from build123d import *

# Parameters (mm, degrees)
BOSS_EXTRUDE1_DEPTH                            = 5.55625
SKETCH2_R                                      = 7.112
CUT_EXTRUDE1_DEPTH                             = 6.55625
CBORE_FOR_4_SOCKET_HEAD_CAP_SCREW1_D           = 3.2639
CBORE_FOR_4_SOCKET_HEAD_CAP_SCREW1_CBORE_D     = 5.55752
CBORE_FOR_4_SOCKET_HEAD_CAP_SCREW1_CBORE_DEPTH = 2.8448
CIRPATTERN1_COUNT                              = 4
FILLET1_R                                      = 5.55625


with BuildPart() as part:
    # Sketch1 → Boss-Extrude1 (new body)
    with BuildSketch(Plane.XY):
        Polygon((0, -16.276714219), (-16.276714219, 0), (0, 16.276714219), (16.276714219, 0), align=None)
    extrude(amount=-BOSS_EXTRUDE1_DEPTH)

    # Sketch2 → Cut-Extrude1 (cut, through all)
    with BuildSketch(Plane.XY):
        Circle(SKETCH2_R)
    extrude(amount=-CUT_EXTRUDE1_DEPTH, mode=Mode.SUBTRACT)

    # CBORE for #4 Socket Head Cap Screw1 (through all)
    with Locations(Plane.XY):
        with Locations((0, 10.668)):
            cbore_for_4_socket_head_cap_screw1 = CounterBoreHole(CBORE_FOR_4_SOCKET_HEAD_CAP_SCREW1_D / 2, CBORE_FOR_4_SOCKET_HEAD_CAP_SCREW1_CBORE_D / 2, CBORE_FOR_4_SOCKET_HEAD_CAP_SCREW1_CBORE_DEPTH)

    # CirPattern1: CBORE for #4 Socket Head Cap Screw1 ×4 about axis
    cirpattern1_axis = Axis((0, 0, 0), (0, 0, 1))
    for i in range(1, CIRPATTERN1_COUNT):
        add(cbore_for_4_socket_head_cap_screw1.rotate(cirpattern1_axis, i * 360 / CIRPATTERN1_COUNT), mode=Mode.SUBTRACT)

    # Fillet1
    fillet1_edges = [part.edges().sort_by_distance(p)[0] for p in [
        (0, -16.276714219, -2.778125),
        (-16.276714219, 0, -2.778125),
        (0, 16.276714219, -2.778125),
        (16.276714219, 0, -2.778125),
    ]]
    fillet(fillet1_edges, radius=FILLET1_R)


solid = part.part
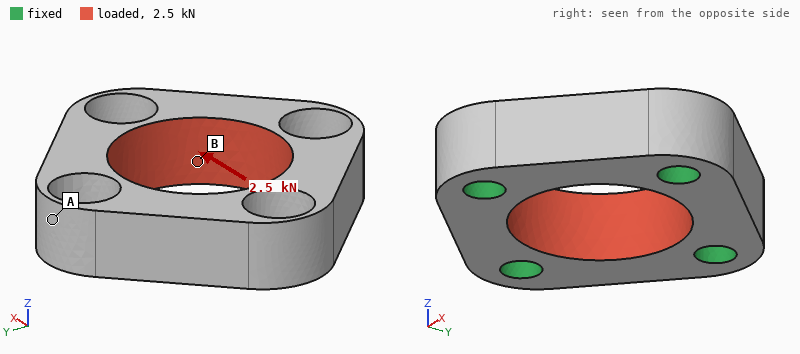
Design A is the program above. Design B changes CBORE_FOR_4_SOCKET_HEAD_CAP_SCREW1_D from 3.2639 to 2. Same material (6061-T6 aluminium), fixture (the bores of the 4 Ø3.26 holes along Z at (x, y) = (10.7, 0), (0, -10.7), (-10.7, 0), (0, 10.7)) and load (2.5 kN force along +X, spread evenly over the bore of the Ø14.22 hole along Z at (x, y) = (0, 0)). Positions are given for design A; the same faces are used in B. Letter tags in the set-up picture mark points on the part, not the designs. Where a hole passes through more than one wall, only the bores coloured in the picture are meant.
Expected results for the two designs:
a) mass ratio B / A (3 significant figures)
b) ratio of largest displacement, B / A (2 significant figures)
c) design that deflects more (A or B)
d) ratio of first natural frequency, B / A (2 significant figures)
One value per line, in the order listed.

1.04
1.2
B
0.78
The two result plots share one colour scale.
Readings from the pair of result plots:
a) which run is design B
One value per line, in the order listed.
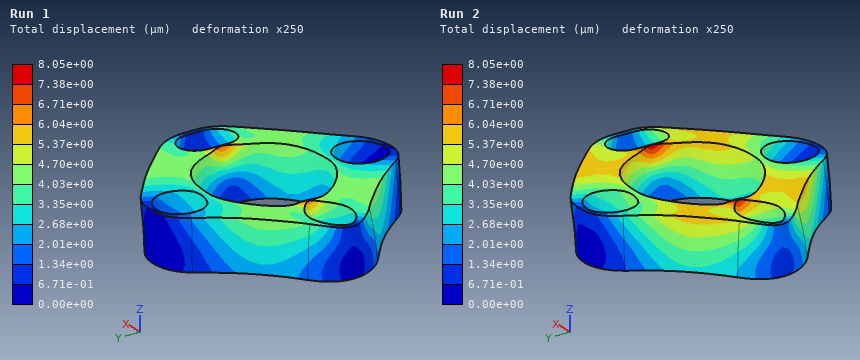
Run 2
